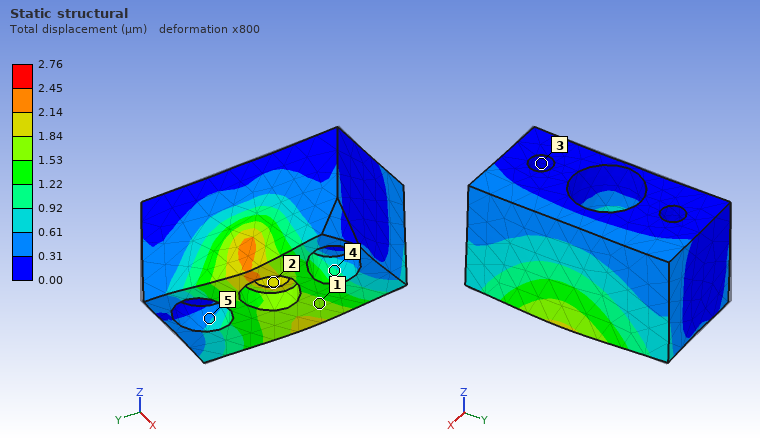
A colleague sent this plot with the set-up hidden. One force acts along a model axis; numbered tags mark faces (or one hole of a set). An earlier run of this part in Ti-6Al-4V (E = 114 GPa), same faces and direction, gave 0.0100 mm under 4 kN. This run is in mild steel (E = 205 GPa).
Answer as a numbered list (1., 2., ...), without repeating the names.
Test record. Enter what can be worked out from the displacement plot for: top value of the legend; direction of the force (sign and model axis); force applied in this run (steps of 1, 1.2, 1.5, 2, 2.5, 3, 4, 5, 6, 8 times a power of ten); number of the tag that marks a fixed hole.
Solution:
1. 2.76 µm
2. +X
3. 2 kN
4. 3
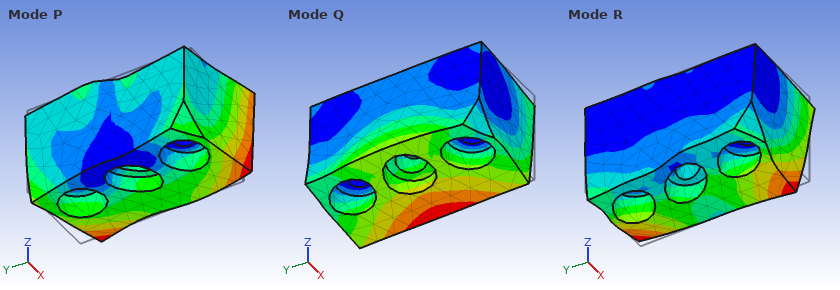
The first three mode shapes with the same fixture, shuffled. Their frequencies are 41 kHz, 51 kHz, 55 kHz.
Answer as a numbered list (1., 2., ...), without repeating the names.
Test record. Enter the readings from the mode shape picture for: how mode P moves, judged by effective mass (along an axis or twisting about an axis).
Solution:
1. along Y
